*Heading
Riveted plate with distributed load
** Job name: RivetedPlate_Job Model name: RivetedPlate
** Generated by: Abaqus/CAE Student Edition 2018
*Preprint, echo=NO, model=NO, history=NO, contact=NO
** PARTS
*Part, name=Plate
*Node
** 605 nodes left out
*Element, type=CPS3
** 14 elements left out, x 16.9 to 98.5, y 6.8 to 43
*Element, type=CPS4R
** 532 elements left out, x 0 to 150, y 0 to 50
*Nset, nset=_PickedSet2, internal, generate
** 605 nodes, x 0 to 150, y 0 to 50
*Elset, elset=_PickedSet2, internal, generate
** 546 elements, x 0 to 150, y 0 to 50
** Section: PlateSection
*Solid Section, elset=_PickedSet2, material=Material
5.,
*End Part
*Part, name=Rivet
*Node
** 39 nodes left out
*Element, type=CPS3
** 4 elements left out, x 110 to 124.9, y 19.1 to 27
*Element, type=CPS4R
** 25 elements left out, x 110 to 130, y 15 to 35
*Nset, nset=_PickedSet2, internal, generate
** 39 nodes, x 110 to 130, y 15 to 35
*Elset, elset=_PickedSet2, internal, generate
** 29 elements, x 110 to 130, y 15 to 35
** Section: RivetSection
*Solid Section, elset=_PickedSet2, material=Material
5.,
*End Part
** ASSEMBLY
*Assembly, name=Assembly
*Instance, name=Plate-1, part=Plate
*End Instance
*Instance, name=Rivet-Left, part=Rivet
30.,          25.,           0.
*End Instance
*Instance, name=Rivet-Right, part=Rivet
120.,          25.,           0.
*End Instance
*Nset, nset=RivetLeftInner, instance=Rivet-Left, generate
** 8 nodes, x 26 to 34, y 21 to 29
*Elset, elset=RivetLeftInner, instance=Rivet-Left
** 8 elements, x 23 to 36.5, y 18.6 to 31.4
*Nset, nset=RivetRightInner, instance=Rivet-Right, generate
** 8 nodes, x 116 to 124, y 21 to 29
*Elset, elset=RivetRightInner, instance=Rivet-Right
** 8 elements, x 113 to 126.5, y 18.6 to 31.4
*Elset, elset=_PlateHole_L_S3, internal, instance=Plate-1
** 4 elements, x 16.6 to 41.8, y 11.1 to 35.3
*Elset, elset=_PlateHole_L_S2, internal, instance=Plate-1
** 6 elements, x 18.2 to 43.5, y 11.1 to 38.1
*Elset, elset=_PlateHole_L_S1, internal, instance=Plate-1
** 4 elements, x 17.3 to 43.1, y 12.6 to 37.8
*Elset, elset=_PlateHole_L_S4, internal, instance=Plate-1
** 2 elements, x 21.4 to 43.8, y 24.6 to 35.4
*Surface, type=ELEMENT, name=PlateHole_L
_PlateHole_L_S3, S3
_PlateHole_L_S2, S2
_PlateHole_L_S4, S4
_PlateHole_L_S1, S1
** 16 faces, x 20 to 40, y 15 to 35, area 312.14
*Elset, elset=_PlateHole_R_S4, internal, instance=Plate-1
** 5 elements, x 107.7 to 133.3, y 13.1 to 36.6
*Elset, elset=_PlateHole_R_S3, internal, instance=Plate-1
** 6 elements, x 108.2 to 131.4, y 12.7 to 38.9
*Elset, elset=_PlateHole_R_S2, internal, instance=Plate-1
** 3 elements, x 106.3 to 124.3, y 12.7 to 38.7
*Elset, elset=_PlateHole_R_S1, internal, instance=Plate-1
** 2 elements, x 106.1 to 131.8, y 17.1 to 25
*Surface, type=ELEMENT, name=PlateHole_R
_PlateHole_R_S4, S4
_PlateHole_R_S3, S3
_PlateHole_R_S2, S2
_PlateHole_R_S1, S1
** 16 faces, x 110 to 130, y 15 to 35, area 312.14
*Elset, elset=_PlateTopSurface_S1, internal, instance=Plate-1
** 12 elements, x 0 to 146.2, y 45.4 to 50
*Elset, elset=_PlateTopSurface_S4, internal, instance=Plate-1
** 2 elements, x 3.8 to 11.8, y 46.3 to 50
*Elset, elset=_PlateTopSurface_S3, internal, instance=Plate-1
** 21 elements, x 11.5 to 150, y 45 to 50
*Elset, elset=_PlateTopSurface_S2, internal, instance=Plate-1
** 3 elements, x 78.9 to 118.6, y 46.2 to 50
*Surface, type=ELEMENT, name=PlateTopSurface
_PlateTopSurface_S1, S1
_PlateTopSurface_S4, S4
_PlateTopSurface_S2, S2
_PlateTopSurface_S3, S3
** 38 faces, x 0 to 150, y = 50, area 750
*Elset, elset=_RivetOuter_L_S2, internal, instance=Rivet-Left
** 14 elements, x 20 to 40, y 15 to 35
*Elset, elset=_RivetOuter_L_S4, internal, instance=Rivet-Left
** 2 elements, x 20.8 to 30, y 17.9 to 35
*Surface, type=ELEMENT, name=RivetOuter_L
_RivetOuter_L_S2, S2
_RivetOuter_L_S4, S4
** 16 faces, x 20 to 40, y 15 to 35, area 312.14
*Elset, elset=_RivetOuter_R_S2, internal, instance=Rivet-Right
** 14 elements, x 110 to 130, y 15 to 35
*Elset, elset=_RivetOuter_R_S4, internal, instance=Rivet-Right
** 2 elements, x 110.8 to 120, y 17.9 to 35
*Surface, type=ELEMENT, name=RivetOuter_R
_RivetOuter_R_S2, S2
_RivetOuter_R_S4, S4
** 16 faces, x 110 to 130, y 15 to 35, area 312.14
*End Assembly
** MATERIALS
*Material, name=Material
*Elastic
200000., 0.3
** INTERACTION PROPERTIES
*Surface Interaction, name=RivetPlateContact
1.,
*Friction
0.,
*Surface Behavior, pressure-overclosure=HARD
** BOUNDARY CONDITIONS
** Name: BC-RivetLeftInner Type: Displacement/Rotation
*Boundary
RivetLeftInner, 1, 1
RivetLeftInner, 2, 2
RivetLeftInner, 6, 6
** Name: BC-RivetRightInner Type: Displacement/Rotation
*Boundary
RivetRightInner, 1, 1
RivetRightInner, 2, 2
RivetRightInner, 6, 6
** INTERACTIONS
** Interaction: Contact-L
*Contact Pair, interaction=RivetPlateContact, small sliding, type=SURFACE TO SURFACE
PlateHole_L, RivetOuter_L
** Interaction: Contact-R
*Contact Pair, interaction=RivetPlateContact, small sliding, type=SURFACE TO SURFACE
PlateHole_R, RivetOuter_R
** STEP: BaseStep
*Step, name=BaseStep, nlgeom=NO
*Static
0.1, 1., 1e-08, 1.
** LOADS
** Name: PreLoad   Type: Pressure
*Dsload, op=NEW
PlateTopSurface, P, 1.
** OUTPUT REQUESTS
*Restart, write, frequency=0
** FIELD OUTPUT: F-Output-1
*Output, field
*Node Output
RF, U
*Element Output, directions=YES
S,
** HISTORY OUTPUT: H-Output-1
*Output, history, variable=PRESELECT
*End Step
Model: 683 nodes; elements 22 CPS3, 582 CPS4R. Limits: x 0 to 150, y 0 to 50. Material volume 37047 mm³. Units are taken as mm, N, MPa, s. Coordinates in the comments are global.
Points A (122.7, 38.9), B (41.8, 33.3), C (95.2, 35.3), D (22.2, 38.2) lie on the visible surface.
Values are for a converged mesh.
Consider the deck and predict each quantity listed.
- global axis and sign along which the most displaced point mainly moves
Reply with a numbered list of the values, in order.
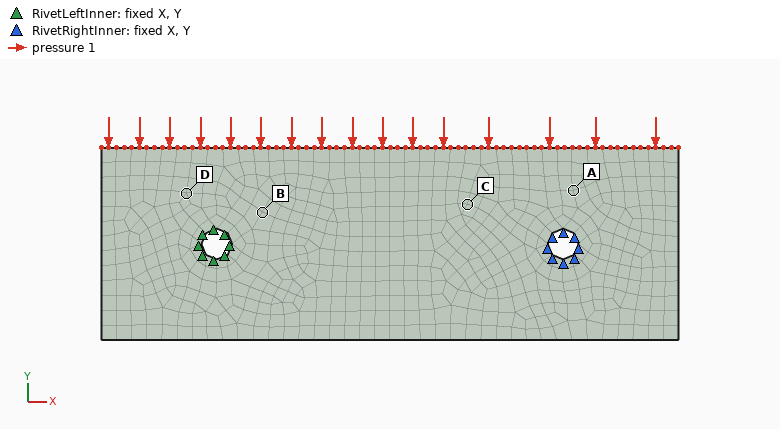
1. -Y
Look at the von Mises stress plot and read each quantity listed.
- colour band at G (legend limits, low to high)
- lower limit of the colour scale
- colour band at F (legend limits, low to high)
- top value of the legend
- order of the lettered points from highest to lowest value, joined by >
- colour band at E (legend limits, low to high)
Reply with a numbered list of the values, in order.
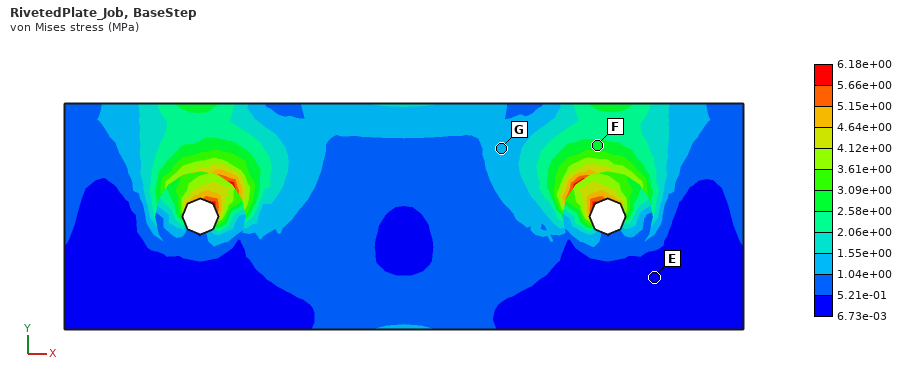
1. 1.04e+00 to 1.55e+00 MPa
2. 6.73e-03 MPa
3. 2.58e+00 to 3.09e+00 MPa
4. 6.18e+00 MPa
5. F > G > E
6. 6.73e-03 to 5.21e-01 MPa
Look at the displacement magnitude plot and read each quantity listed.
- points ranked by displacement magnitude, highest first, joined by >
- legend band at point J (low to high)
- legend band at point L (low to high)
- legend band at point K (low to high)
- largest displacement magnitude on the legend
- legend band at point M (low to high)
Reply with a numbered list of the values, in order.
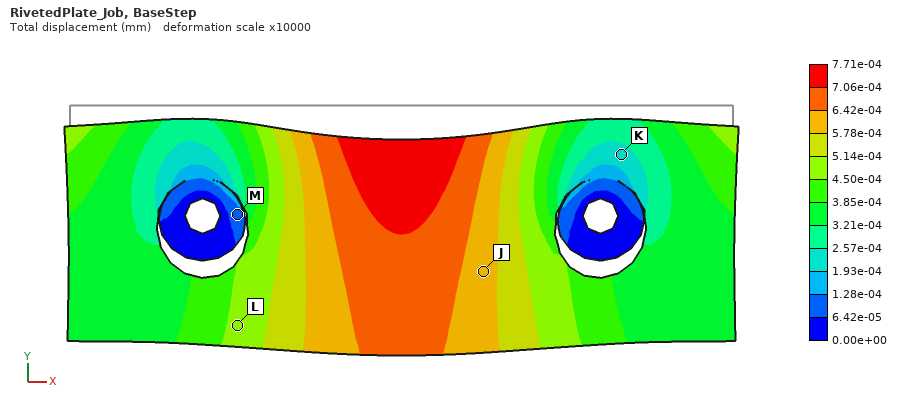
1. J > L > K > M
2. 5.78e-04 to 6.42e-04 mm
3. 4.50e-04 to 5.14e-04 mm
4. 1.93e-04 to 2.57e-04 mm
5. 7.71e-04 mm
6. 6.42e-05 to 1.28e-04 mm
